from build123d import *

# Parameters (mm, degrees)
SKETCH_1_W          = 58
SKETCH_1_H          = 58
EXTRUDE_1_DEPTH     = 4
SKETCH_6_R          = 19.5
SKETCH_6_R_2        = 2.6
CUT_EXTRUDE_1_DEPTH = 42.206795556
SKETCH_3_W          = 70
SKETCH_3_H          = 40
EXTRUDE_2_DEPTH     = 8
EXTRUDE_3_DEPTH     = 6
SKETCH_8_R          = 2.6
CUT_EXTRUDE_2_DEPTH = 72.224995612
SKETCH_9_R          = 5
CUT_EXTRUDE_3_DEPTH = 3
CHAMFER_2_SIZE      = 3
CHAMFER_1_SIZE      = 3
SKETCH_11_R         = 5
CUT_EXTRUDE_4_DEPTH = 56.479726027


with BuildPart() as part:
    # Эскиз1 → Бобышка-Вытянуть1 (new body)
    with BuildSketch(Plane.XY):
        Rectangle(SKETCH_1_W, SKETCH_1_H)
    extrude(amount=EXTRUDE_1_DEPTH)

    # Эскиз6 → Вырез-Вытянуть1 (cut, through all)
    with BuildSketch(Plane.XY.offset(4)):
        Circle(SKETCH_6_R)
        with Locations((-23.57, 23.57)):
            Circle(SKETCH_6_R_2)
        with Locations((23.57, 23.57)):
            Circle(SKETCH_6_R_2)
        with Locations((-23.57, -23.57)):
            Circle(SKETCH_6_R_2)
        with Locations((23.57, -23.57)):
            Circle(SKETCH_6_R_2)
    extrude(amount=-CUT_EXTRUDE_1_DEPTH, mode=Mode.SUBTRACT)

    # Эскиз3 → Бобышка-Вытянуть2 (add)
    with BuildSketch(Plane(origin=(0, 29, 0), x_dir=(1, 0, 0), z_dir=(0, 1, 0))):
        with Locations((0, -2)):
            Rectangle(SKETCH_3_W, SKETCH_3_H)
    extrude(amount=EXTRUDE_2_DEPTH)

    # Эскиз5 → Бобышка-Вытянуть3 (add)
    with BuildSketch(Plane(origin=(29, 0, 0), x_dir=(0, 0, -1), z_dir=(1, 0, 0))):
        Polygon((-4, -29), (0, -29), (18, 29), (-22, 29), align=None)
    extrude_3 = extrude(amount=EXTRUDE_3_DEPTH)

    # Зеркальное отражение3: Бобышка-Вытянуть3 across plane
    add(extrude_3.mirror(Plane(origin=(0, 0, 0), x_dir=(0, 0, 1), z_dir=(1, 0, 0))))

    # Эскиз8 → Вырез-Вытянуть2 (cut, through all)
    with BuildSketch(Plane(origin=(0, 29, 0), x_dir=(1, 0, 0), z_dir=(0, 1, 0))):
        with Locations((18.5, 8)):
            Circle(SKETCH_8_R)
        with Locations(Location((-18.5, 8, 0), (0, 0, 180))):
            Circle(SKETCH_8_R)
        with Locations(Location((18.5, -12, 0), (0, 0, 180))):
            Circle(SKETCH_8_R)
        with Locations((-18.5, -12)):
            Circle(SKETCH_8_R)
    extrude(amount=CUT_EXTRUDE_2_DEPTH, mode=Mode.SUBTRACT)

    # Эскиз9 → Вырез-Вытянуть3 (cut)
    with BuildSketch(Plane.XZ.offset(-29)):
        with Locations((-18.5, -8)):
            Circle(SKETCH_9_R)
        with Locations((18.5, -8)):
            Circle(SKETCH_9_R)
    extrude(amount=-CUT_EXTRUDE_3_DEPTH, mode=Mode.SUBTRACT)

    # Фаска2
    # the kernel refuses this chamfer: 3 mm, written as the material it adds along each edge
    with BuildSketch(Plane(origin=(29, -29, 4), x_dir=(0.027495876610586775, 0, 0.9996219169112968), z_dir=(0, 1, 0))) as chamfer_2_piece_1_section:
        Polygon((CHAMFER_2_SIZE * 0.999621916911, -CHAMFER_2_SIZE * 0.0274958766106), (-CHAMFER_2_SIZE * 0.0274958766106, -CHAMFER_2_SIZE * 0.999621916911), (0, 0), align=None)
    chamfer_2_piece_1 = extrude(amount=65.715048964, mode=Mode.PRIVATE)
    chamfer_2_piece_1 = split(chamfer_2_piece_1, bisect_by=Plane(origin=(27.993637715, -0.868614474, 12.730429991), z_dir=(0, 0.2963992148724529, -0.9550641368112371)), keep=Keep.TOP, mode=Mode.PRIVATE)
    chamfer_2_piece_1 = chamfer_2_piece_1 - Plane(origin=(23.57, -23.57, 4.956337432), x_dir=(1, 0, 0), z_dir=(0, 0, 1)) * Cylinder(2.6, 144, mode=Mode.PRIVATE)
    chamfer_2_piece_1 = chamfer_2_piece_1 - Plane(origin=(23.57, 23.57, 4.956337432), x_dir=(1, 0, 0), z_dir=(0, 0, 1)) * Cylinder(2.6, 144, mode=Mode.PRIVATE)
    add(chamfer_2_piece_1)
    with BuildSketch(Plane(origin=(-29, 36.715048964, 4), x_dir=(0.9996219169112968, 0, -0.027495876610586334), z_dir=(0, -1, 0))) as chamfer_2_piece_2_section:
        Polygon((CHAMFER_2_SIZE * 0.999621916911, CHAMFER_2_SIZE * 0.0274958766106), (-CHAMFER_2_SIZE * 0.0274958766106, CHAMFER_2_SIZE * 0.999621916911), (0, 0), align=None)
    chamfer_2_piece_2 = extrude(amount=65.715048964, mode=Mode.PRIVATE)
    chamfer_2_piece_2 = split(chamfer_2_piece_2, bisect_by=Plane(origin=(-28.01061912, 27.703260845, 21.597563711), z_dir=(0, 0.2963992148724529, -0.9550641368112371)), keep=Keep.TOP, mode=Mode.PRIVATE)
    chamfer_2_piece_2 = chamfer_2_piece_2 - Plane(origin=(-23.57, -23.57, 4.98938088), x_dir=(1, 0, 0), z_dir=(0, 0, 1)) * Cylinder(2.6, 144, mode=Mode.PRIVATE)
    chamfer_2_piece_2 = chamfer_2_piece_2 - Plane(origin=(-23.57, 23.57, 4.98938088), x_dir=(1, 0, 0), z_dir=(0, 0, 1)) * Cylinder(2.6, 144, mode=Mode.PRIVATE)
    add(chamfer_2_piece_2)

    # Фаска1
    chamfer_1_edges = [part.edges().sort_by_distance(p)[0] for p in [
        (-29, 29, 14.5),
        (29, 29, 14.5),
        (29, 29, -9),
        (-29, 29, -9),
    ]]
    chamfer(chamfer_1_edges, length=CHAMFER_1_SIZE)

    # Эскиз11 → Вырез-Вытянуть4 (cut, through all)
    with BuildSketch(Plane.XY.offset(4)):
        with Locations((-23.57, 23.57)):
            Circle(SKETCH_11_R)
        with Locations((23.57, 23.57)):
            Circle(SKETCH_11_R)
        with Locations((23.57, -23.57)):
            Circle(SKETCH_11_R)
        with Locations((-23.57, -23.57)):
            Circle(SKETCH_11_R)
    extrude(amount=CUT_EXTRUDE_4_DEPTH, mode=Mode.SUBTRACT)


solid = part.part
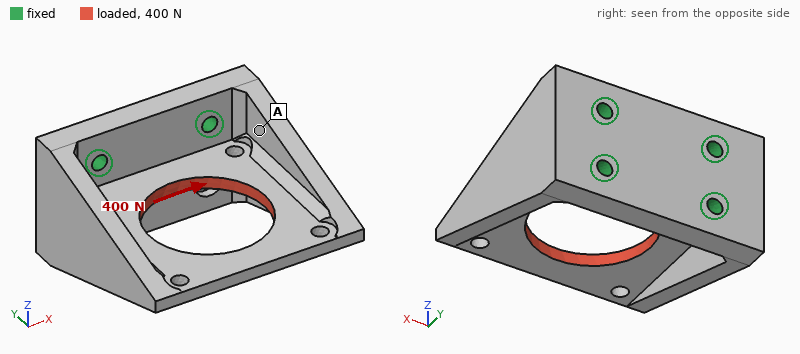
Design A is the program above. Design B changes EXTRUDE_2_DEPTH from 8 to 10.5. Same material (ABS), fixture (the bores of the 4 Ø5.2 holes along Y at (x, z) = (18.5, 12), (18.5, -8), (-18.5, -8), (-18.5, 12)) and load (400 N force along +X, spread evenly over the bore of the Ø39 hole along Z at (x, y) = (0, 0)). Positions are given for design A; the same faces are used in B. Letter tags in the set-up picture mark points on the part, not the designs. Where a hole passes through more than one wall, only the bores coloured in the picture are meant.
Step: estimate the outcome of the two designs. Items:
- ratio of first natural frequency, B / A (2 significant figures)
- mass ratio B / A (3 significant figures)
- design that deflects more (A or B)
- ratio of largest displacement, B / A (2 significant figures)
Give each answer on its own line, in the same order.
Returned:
1.1
1.15
A
0.84
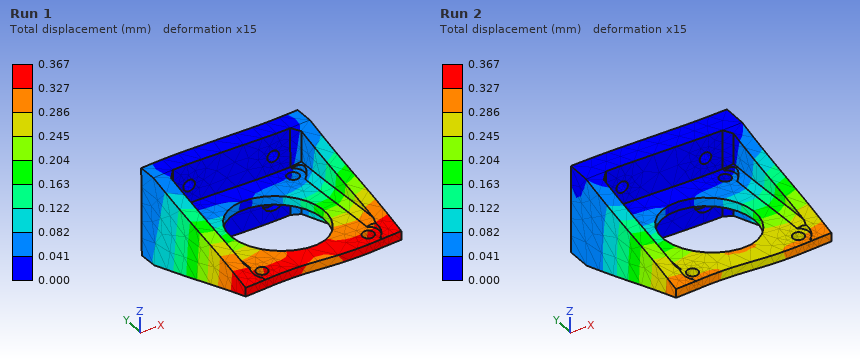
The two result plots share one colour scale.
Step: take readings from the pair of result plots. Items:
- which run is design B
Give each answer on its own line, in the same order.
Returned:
Run 2
